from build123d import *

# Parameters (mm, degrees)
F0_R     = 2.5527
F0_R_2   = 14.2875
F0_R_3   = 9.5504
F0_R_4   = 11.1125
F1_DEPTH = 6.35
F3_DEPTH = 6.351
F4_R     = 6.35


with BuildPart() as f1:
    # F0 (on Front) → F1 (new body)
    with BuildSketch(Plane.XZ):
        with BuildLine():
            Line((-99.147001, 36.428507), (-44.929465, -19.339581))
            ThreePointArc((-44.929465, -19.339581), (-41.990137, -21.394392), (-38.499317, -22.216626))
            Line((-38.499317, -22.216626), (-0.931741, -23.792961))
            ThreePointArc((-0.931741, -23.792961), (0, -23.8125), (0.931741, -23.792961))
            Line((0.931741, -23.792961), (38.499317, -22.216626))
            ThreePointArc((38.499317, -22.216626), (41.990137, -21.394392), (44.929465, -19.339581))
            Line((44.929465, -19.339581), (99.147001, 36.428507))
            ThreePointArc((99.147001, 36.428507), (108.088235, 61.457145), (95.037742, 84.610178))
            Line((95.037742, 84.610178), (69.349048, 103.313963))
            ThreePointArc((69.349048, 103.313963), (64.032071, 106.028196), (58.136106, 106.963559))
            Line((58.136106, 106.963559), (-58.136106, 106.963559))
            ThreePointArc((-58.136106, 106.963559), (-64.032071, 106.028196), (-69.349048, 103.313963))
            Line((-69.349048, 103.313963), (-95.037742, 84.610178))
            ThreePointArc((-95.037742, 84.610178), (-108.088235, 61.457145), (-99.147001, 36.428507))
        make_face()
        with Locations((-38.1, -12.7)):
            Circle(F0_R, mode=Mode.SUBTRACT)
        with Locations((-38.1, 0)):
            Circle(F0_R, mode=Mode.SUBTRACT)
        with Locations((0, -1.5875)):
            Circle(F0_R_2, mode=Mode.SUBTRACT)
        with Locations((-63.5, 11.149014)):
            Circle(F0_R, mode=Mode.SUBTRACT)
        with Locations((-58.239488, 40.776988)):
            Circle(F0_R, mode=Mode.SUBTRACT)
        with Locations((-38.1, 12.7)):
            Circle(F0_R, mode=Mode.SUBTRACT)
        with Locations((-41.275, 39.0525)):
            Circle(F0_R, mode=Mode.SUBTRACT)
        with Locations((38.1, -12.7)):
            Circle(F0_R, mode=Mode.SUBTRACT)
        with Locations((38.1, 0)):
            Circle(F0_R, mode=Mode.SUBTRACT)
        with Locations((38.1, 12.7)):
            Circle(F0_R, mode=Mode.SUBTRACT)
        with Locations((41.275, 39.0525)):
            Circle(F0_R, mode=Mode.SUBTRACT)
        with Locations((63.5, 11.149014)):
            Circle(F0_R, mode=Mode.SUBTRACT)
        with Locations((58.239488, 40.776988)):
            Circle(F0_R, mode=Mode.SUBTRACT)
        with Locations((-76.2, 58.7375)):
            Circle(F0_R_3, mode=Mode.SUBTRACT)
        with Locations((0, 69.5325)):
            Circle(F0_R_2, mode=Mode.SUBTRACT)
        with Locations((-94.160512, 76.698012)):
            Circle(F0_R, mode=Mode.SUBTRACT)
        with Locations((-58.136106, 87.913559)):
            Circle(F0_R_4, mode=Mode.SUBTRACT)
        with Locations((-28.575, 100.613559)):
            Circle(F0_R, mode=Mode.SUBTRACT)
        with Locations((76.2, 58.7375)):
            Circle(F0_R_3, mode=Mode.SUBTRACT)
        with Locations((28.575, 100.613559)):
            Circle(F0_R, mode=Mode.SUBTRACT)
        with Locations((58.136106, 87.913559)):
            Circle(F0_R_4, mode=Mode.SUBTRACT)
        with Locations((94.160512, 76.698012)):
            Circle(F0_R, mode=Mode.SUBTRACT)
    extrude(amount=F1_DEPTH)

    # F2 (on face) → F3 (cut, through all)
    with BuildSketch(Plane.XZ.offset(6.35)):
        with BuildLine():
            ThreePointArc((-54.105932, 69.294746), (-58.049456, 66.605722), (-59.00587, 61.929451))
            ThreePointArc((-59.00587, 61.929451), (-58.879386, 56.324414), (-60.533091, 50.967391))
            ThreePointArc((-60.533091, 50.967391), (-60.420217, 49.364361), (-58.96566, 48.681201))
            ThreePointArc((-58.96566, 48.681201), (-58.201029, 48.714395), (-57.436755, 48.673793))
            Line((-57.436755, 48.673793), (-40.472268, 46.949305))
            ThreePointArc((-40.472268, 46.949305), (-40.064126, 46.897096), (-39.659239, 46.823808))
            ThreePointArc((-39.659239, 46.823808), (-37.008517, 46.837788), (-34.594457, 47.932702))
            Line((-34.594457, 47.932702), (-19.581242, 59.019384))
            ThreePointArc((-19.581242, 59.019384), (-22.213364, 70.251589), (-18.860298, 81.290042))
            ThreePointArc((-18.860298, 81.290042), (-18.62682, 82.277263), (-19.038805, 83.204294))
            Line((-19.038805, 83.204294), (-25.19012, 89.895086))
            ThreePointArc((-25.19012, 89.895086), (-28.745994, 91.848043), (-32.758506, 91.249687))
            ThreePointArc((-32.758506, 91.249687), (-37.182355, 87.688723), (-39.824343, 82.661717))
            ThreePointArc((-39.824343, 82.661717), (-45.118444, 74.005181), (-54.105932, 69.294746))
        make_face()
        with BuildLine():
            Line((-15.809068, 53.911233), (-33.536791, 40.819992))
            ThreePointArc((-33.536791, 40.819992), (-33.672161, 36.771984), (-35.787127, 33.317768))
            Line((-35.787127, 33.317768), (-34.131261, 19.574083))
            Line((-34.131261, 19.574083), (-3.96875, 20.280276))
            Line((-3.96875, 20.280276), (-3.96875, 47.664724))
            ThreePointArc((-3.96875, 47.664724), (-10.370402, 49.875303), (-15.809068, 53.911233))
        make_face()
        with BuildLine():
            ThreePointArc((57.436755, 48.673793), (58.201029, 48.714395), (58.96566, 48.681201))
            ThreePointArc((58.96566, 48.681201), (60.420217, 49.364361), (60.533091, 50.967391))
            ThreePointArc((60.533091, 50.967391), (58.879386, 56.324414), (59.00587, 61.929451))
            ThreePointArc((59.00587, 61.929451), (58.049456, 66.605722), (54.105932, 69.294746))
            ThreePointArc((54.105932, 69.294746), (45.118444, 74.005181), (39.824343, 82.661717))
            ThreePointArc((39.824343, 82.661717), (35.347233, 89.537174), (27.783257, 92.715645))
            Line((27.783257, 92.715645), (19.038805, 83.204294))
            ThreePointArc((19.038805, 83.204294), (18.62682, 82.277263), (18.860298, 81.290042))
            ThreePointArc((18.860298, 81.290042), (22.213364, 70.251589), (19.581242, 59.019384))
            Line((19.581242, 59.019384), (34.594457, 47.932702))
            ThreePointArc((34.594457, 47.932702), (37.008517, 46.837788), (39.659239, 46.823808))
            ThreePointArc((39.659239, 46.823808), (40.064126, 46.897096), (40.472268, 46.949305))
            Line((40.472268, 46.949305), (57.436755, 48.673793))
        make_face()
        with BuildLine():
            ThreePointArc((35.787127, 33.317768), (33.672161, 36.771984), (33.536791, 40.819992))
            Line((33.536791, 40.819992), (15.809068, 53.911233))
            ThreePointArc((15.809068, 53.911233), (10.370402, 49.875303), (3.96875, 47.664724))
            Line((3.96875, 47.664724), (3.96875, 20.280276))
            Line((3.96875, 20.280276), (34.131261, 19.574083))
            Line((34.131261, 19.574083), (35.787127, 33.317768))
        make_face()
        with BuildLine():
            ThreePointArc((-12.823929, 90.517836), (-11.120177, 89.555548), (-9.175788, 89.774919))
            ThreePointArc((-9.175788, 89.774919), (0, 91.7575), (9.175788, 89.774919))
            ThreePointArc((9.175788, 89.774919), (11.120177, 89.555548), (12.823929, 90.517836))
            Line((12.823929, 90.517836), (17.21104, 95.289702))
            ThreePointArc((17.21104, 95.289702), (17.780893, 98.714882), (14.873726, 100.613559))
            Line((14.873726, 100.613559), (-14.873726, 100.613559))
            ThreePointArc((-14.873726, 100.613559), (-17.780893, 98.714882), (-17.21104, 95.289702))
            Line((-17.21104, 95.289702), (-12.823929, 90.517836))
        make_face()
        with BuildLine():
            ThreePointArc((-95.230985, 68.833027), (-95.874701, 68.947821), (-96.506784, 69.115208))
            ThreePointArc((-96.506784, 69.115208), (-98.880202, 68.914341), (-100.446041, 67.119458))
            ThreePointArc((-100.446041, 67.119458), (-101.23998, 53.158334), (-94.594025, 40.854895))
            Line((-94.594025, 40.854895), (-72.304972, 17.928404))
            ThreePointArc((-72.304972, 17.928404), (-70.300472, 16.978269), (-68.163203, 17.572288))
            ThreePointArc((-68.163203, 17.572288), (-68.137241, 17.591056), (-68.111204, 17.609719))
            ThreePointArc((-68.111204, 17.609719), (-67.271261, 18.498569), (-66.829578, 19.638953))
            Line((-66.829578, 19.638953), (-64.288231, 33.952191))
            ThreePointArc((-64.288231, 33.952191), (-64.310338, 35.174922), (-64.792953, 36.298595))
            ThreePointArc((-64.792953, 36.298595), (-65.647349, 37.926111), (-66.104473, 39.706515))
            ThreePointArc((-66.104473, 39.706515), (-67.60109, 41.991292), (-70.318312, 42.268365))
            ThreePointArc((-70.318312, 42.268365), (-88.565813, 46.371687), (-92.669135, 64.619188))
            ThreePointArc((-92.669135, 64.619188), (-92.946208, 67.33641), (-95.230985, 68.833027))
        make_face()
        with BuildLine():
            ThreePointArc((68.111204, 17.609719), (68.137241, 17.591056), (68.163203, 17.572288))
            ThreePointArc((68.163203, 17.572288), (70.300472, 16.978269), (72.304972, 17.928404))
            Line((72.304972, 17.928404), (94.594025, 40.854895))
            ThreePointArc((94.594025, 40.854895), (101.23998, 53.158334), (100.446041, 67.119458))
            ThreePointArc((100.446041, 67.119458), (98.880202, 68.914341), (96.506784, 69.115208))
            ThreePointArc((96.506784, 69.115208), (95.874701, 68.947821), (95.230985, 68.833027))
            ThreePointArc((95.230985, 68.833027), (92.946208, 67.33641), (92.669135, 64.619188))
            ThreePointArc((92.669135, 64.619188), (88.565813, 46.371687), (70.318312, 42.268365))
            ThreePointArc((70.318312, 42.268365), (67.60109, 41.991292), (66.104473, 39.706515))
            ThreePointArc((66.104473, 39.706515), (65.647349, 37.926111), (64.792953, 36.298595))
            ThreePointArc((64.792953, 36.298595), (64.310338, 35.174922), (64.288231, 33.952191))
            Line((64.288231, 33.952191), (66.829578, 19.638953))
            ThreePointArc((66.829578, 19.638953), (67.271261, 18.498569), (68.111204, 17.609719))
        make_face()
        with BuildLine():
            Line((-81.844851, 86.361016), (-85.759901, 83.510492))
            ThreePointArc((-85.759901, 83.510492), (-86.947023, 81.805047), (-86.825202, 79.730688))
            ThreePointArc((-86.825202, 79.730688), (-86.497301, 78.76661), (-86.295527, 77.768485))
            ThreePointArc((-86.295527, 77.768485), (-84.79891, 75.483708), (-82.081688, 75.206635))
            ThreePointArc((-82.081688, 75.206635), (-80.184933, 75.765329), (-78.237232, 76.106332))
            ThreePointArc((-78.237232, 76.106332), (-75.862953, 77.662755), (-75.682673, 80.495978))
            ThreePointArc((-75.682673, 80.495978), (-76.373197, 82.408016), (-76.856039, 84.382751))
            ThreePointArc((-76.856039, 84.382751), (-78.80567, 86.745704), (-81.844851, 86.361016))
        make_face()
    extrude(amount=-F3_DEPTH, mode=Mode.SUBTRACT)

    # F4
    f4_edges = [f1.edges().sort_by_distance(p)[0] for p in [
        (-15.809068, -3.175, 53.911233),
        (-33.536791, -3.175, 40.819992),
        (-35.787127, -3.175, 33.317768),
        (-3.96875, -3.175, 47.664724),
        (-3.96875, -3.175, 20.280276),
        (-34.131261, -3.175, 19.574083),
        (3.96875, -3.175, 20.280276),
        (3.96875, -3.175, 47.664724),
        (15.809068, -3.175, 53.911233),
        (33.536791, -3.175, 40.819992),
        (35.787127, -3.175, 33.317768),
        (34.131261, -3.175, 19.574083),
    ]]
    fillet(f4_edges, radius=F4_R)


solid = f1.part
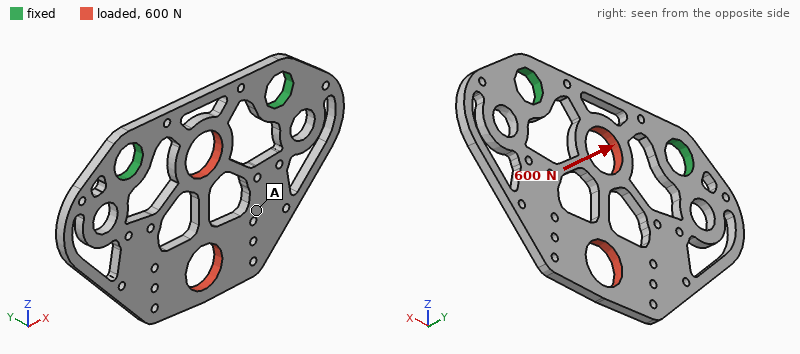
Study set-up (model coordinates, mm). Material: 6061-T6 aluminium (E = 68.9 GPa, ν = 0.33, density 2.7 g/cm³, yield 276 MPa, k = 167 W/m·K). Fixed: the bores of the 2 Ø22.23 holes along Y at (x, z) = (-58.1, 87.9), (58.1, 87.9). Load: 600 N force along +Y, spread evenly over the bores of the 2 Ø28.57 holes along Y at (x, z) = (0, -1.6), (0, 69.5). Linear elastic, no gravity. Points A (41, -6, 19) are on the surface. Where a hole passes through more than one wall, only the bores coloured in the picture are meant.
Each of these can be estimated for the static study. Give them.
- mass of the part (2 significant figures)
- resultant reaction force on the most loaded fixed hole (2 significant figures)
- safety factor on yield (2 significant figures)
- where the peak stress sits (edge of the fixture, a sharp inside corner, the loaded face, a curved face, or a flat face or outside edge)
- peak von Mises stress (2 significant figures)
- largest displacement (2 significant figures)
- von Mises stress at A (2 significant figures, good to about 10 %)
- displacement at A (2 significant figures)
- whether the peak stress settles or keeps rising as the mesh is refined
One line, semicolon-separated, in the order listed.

230 g; 300 N; 1.8; a curved face; 160 MPa; 1.4 mm; 11 MPa; 0.64 mm; settles
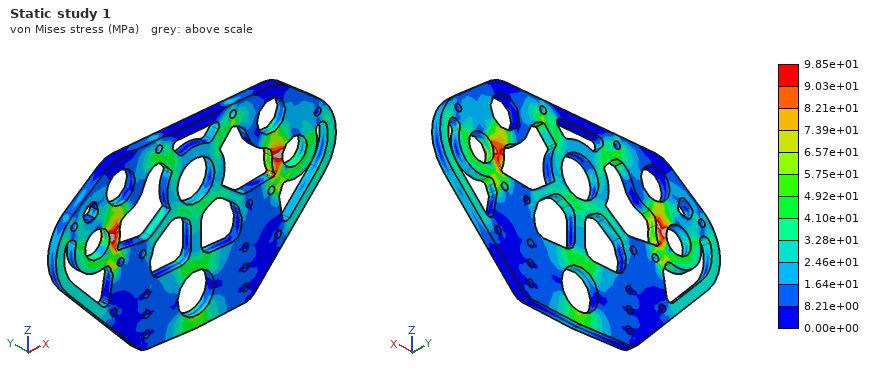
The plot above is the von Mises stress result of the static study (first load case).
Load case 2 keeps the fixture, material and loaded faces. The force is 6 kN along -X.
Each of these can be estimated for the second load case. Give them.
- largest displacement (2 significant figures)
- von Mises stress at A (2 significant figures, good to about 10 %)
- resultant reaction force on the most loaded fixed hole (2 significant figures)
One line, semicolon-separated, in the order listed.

0.13 mm; 15 MPa; 3.6 kN
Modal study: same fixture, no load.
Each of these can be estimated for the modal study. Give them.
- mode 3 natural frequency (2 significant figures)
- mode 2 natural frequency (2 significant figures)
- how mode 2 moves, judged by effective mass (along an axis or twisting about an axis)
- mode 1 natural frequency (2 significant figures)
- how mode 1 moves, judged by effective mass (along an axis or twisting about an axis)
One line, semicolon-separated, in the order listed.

1700 Hz; 910 Hz; twisting about Z; 340 Hz; along Y
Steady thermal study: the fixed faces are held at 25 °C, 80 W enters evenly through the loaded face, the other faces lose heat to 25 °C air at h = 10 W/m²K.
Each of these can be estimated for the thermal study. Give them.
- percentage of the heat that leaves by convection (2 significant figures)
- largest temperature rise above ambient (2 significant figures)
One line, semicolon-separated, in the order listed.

18 %; 77 K
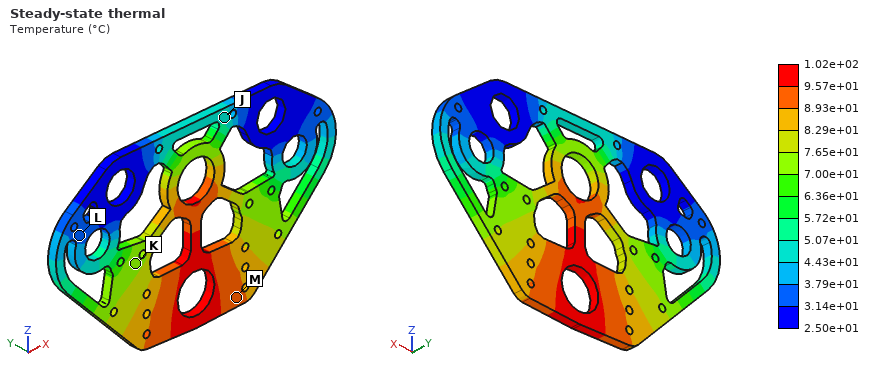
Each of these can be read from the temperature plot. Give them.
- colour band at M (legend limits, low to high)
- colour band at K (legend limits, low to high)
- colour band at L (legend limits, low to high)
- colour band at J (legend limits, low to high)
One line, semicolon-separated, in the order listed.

8.93e+01 to 9.57e+01 °C; 7.00e+01 to 7.65e+01 °C; 3.14e+01 to 3.79e+01 °C; 4.43e+01 to 5.07e+01 °C
